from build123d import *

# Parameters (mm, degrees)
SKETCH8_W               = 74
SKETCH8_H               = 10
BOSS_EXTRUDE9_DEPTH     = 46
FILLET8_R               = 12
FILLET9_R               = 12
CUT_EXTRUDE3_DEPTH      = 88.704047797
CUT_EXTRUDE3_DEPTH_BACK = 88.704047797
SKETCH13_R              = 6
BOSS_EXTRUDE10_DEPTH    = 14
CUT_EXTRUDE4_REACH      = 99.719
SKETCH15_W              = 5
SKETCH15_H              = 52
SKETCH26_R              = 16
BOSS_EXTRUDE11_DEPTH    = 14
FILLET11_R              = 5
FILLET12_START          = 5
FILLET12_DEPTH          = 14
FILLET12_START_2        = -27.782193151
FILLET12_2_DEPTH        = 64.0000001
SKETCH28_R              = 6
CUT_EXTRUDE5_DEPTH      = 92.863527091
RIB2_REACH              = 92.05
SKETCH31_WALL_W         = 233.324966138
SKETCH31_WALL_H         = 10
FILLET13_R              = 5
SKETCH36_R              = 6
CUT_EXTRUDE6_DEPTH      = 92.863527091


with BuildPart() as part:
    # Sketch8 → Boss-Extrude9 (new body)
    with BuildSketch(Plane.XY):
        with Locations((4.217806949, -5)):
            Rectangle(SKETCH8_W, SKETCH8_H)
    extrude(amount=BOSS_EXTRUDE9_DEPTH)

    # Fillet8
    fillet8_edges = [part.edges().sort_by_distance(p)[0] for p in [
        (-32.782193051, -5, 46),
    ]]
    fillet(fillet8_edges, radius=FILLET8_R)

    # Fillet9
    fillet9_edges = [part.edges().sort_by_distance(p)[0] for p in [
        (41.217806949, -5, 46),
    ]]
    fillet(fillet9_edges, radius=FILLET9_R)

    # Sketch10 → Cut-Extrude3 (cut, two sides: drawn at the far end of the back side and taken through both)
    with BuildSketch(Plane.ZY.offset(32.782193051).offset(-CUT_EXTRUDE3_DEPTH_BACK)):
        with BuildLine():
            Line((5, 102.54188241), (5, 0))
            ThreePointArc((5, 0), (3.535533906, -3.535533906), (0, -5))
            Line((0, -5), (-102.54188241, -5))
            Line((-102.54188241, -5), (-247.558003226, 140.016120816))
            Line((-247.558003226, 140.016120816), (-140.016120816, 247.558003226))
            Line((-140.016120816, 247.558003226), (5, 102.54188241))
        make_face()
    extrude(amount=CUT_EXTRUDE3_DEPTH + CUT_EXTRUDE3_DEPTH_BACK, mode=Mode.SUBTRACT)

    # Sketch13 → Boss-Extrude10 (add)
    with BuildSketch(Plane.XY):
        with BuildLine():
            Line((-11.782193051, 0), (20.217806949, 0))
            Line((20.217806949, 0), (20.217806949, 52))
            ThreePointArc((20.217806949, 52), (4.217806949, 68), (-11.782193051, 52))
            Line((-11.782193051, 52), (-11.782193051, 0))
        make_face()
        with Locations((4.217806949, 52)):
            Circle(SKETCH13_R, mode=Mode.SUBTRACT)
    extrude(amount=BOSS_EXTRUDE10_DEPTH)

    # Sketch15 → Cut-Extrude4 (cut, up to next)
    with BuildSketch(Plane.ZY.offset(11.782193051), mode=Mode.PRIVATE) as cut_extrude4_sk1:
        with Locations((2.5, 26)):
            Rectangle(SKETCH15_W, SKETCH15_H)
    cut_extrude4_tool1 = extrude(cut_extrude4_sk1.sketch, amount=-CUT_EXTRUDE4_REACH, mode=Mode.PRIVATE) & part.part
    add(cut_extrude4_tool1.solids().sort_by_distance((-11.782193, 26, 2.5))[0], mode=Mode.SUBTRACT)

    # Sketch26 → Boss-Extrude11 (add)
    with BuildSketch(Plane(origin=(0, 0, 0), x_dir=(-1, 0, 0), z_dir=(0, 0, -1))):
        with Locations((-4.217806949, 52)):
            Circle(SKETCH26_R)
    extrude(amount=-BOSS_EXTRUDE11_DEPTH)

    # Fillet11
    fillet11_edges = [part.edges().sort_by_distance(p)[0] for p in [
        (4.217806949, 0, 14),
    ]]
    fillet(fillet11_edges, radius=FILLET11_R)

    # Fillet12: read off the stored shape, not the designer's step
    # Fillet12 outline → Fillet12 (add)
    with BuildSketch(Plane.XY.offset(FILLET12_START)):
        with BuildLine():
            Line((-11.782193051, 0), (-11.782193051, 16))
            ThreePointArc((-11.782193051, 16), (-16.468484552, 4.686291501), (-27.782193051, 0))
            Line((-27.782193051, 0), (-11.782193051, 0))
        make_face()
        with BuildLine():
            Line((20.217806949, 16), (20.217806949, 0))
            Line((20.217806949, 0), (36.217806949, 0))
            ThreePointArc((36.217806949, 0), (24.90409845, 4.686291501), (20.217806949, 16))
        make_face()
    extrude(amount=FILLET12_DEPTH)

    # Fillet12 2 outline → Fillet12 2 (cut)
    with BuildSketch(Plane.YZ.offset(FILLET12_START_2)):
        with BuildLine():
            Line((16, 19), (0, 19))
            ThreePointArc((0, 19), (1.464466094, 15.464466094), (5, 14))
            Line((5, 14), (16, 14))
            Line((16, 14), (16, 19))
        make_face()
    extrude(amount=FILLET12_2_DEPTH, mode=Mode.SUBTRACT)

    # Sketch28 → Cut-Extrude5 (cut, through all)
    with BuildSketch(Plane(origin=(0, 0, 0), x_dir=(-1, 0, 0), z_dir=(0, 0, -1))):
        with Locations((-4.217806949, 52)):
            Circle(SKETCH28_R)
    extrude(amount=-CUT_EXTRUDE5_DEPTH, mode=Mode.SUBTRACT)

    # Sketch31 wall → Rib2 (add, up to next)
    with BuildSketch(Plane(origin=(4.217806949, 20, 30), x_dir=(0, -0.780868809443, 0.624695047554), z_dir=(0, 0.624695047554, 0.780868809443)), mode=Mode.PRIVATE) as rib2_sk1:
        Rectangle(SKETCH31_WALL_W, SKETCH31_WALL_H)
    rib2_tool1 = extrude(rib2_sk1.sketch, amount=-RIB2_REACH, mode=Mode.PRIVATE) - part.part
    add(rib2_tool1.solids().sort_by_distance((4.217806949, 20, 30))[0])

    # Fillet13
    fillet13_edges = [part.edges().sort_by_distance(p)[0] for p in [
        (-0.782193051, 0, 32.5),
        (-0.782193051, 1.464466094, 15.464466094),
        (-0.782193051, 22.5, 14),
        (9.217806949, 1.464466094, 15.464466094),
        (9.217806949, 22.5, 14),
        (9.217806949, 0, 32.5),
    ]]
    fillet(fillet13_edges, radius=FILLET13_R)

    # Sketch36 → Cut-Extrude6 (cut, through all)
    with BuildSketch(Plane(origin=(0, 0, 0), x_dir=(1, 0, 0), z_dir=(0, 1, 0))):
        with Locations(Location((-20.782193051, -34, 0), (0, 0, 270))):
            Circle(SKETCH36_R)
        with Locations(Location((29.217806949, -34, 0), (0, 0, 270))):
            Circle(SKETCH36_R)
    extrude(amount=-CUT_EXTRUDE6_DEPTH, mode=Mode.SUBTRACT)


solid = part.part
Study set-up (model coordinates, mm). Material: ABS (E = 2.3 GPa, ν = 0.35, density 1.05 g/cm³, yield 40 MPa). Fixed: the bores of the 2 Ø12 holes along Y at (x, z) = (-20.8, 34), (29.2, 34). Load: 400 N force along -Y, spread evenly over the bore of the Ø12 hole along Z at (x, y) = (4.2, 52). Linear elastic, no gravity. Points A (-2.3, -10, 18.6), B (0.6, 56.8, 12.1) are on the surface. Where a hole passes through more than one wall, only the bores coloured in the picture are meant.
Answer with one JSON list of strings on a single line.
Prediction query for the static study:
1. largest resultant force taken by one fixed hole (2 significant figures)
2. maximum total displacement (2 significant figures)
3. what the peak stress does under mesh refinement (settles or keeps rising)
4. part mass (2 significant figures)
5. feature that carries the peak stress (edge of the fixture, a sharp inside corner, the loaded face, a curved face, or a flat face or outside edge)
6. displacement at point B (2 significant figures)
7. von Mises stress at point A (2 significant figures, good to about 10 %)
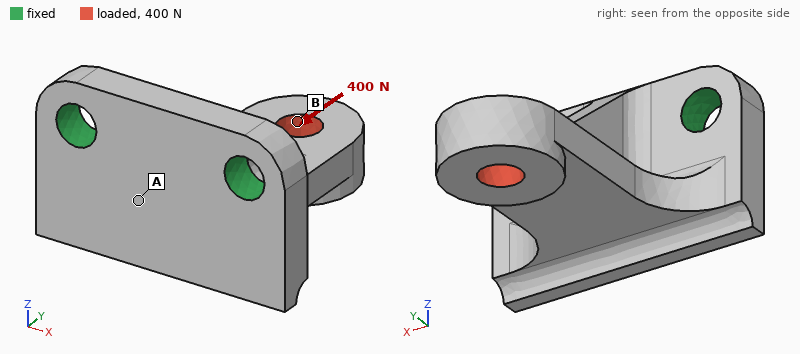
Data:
["200 N", "0.60 mm", "keeps rising", "62 g", "edge of the fixture", "0.46 mm", "1.9 MPa"]
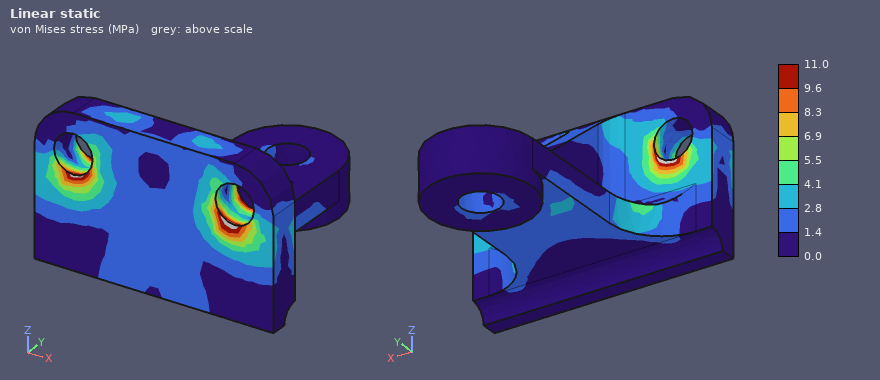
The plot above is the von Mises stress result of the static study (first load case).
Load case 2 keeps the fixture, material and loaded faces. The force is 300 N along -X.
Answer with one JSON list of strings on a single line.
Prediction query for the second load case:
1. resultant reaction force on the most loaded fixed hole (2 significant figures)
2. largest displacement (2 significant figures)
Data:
["430 N", "0.69 mm"]
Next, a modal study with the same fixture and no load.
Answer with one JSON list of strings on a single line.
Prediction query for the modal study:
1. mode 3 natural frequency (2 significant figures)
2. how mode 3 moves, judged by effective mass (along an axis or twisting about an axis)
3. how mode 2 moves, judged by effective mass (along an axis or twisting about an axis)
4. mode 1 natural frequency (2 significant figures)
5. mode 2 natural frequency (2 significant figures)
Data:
["2000 Hz", "along Y", "along X", "700 Hz", "1100 Hz"]
